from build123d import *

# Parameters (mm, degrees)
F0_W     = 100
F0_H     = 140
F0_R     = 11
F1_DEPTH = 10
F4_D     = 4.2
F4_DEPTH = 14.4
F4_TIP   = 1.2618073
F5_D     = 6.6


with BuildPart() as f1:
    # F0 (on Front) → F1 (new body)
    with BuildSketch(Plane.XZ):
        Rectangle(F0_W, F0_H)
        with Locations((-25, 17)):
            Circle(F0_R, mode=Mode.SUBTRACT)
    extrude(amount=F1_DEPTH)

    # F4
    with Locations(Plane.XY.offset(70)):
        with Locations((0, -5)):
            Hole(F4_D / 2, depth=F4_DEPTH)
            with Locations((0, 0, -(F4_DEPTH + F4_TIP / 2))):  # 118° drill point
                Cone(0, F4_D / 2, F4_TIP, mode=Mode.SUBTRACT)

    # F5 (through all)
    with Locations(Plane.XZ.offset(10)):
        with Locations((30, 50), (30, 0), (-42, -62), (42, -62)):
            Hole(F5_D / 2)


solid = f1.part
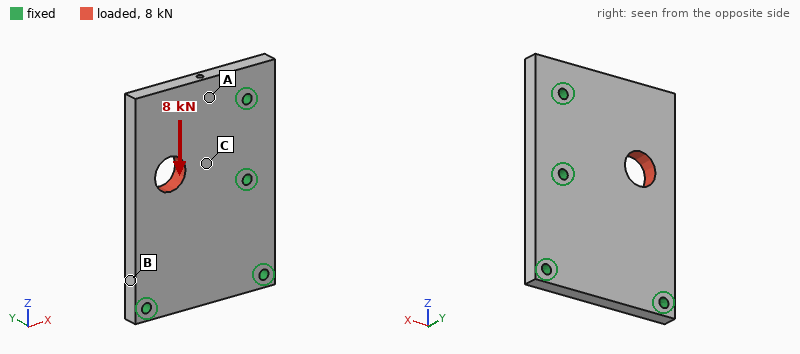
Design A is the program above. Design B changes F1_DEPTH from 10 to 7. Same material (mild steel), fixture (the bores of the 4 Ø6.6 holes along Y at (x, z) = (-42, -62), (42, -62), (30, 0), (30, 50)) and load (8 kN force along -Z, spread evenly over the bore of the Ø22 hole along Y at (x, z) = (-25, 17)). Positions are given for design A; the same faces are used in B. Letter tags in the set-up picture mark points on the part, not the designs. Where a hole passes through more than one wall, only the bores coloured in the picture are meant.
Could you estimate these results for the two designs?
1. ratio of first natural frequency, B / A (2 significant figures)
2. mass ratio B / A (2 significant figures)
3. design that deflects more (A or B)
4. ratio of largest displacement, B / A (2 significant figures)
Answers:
0.72
0.70
B
1.5
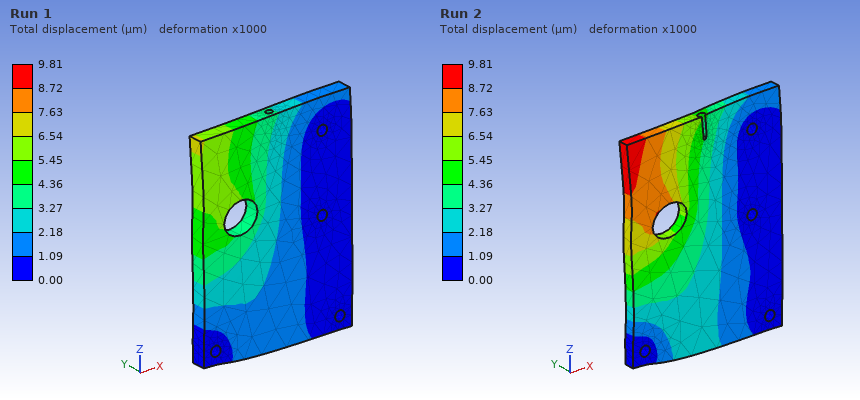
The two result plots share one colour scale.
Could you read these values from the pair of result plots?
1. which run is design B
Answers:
Run 2
